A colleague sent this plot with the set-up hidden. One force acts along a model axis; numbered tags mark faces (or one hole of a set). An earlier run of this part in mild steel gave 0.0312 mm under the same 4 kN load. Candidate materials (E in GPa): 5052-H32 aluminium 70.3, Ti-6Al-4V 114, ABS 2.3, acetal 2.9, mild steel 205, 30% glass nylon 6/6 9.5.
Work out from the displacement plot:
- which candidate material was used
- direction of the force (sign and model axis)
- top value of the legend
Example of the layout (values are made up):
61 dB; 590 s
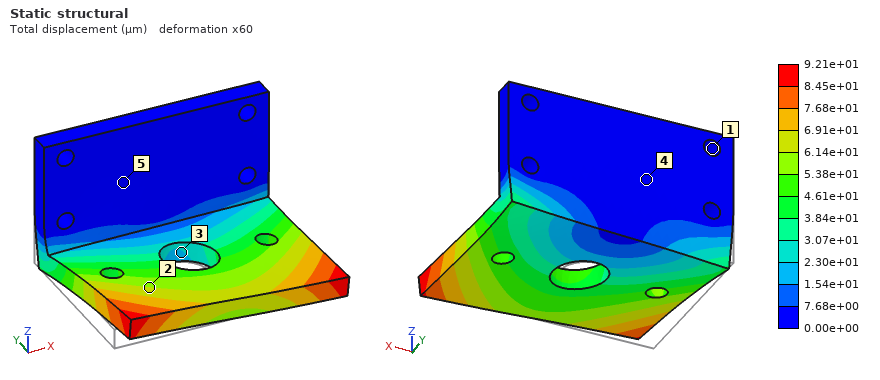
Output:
5052-H32 aluminium; +X; 9.21e+01 µm
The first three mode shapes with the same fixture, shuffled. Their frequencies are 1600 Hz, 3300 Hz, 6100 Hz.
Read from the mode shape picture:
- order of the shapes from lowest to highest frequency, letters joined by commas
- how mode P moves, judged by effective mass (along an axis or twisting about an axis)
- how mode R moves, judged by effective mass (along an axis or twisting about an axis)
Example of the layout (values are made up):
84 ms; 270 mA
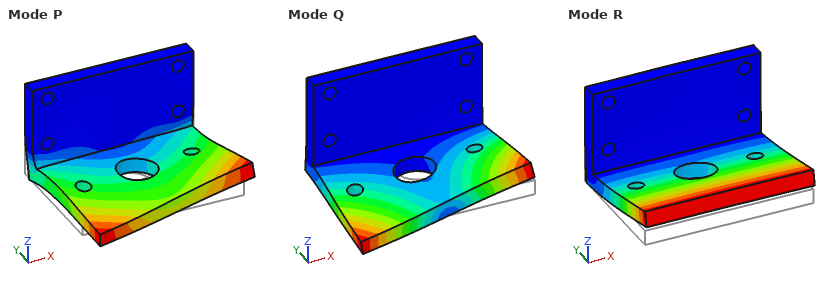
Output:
R, Q, P; along X; along Z
